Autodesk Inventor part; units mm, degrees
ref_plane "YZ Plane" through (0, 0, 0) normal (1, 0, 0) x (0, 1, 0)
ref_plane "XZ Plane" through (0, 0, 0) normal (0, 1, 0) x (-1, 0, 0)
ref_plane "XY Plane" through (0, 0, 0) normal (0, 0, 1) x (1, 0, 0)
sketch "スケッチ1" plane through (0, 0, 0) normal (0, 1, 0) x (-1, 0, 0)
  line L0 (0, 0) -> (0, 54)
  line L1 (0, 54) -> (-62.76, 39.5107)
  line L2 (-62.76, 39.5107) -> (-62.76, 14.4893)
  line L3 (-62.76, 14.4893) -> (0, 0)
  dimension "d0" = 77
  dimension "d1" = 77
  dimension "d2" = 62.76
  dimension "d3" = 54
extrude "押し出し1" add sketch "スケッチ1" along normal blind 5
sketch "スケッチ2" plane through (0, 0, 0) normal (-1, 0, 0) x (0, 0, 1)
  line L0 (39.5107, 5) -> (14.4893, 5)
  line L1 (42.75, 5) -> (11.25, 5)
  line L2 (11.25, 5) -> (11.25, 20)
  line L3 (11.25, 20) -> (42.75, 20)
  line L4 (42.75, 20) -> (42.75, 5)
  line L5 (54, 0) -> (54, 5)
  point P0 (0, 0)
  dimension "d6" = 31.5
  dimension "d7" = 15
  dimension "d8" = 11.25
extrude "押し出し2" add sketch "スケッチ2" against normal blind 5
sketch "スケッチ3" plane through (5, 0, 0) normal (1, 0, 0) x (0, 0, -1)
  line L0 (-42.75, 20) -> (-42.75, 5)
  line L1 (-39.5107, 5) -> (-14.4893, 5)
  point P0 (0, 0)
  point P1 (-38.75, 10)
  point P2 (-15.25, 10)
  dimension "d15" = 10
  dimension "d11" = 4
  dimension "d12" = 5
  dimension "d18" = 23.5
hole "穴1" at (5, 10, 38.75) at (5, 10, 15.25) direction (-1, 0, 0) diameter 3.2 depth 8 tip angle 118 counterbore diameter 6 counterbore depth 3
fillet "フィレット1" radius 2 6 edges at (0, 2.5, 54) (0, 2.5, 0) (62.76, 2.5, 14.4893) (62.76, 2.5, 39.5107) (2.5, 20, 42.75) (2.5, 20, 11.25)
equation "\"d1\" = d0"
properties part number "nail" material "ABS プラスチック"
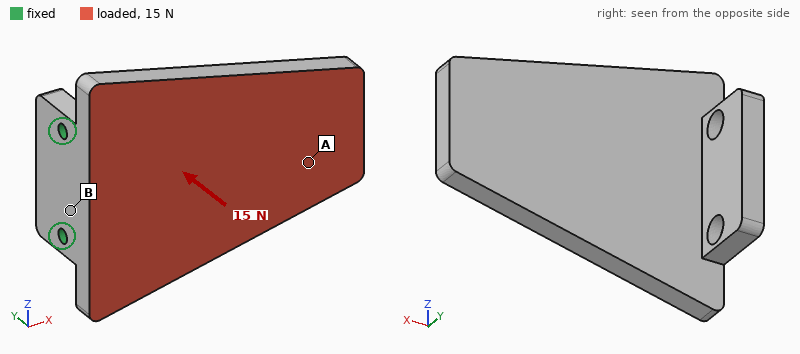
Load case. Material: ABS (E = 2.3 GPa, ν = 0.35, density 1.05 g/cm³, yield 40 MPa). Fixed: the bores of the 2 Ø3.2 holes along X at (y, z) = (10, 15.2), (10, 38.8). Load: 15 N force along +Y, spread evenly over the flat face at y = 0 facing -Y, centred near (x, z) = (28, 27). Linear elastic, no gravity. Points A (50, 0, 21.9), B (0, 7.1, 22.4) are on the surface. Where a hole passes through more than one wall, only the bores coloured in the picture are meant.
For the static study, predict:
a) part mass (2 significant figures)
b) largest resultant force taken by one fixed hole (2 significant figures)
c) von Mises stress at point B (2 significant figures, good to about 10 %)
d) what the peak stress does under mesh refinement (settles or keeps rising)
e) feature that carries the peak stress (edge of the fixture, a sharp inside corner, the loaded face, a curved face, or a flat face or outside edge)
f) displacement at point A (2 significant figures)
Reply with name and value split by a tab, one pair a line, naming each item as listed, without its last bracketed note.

part mass	15 g
largest resultant force taken by one fixed hole	7.8 N
von Mises stress at point B	2.4 MPa
what the peak stress does under mesh refinement	keeps rising
feature that carries the peak stress	edge of the fixture
displacement at point A	0.74 mm
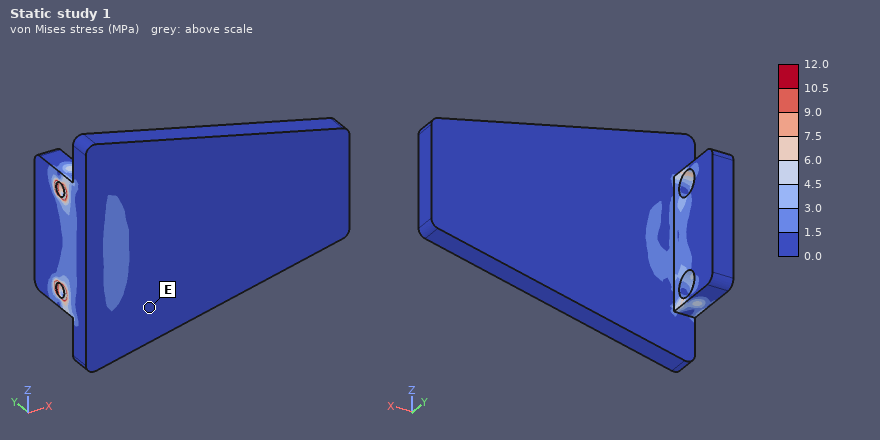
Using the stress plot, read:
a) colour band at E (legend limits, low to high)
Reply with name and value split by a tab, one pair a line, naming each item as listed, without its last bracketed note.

colour band at E	0.0 to 1.5 MPa
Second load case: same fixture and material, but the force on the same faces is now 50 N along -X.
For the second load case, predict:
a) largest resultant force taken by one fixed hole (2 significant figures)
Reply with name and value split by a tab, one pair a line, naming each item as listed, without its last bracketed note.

largest resultant force taken by one fixed hole	25 N
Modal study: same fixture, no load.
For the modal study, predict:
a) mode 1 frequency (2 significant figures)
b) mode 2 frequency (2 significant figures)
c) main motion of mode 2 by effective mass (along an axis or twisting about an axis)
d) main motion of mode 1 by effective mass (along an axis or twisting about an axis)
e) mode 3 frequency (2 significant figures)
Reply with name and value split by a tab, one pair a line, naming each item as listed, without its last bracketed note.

mode 1 frequency	220 Hz
mode 2 frequency	780 Hz
main motion of mode 2 by effective mass	along Z
main motion of mode 1 by effective mass	along Y
mode 3 frequency	1300 Hz
